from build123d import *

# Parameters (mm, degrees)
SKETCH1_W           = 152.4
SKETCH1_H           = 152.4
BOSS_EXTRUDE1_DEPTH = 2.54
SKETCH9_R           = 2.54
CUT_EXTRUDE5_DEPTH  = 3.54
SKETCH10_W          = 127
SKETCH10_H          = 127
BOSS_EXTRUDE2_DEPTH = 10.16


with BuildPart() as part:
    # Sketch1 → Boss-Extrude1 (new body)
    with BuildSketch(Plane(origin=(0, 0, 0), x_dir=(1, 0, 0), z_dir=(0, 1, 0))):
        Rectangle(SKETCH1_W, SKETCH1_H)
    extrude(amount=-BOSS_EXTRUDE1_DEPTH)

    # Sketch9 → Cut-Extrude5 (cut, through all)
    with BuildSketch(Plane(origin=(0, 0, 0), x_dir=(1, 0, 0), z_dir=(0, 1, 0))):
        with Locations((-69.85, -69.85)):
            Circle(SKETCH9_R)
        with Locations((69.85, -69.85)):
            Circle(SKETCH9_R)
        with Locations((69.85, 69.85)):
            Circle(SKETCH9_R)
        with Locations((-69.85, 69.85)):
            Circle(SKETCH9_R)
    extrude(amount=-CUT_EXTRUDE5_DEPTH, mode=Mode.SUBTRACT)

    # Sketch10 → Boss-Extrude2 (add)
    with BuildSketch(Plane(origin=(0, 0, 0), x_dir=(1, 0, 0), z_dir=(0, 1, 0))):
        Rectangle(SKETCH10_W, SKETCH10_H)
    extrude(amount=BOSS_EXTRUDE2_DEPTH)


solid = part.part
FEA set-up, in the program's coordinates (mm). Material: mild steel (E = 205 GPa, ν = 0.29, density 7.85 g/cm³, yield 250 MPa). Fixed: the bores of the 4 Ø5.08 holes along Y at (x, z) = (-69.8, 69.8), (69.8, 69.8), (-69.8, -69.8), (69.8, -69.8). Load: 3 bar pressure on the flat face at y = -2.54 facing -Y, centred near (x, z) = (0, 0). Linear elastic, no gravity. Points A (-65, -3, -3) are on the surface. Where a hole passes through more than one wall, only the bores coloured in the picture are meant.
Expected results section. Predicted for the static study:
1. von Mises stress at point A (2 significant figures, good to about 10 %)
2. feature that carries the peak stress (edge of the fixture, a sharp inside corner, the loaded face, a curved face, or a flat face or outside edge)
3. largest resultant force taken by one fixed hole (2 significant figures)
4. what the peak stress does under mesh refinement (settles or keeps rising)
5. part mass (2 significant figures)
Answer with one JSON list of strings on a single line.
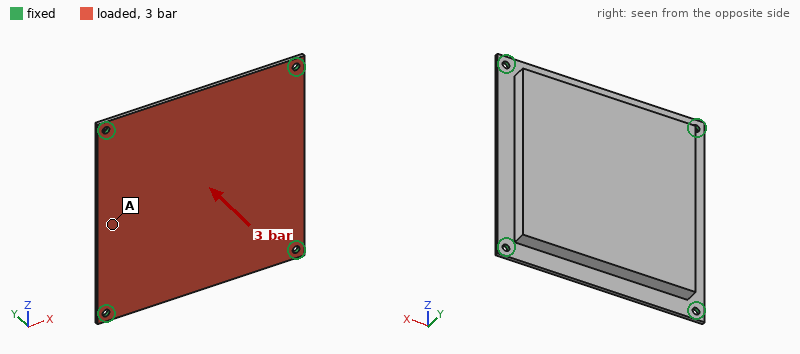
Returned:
["28 MPa", "edge of the fixture", "3.2 kN", "keeps rising", "1.7 kg"]
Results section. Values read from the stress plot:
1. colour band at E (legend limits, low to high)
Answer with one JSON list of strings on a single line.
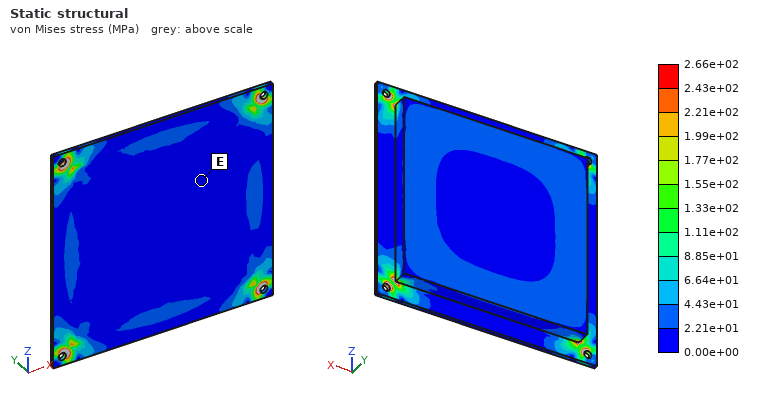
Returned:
["0.00e+00 to 2.21e+01 MPa"]
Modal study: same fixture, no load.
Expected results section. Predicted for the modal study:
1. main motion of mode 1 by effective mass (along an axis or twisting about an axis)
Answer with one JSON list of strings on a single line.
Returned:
["along Y"]
